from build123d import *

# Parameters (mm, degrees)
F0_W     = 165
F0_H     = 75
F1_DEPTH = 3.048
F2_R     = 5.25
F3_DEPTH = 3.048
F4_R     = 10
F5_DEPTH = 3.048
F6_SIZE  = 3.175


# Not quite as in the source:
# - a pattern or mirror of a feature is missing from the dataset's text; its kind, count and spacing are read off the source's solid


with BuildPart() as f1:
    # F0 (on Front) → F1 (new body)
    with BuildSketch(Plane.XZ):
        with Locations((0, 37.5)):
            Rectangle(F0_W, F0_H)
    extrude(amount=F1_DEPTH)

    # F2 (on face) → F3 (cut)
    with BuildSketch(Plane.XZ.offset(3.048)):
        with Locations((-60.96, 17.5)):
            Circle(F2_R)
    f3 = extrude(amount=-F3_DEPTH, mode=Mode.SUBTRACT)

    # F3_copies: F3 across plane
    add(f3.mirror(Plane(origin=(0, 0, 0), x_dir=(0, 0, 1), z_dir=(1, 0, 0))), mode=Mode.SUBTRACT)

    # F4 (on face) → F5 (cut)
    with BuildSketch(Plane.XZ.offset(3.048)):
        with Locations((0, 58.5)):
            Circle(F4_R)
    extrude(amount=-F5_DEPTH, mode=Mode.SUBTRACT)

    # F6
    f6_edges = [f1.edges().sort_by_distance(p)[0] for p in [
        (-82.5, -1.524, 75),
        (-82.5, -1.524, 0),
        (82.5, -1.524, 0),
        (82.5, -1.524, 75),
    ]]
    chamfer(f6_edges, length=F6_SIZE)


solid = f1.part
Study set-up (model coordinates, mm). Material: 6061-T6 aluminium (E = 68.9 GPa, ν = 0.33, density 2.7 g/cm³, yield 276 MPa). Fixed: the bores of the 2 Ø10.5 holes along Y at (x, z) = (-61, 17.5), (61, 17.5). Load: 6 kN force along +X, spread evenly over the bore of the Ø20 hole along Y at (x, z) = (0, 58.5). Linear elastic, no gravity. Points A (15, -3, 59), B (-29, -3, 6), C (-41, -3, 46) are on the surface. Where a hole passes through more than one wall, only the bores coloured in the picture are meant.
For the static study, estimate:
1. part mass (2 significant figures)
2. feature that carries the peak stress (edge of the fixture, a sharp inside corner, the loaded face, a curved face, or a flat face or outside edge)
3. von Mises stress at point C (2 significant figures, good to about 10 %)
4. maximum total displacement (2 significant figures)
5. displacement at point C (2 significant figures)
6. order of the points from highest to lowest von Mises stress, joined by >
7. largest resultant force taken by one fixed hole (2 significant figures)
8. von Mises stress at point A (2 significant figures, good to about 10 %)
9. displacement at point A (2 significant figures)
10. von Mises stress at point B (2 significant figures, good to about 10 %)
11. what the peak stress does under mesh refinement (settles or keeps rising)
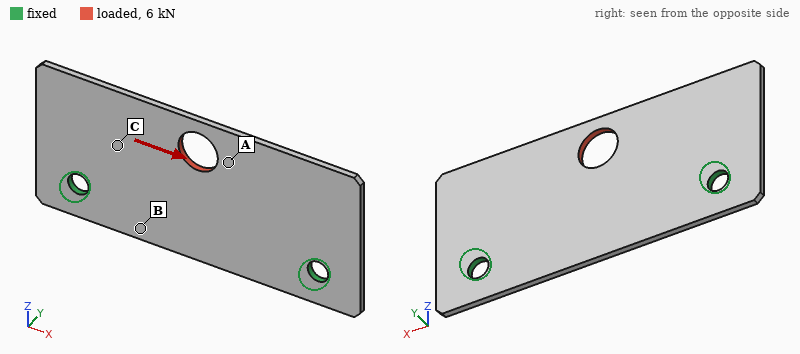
98 g
edge of the fixture
24 MPa
48 µm
21 µm
A > C > B
3.5 kN
38 MPa
35 µm
11 MPa
keeps rising
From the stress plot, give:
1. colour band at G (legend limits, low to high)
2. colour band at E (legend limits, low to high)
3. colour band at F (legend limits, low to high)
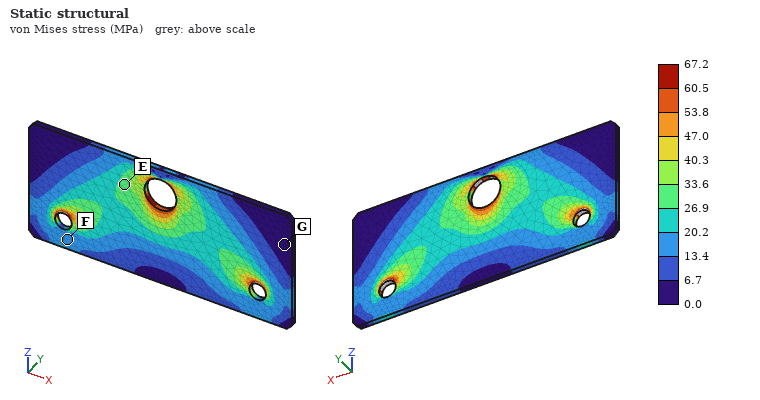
0.0 to 6.7 MPa
26.9 to 33.6 MPa
13.4 to 20.2 MPa
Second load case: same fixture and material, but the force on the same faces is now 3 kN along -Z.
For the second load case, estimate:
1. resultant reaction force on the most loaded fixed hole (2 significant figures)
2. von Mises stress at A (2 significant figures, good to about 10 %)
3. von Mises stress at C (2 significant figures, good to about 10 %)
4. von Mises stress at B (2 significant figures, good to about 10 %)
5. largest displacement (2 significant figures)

1.7 kN
23 MPa
14 MPa
7.7 MPa
37 µm
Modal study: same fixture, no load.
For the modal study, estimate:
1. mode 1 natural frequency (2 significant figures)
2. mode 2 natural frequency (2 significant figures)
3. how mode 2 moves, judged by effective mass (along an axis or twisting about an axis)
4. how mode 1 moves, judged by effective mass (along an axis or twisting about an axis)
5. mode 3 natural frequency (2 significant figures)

620 Hz
1000 Hz
twisting about Z
along Y
1100 Hz
